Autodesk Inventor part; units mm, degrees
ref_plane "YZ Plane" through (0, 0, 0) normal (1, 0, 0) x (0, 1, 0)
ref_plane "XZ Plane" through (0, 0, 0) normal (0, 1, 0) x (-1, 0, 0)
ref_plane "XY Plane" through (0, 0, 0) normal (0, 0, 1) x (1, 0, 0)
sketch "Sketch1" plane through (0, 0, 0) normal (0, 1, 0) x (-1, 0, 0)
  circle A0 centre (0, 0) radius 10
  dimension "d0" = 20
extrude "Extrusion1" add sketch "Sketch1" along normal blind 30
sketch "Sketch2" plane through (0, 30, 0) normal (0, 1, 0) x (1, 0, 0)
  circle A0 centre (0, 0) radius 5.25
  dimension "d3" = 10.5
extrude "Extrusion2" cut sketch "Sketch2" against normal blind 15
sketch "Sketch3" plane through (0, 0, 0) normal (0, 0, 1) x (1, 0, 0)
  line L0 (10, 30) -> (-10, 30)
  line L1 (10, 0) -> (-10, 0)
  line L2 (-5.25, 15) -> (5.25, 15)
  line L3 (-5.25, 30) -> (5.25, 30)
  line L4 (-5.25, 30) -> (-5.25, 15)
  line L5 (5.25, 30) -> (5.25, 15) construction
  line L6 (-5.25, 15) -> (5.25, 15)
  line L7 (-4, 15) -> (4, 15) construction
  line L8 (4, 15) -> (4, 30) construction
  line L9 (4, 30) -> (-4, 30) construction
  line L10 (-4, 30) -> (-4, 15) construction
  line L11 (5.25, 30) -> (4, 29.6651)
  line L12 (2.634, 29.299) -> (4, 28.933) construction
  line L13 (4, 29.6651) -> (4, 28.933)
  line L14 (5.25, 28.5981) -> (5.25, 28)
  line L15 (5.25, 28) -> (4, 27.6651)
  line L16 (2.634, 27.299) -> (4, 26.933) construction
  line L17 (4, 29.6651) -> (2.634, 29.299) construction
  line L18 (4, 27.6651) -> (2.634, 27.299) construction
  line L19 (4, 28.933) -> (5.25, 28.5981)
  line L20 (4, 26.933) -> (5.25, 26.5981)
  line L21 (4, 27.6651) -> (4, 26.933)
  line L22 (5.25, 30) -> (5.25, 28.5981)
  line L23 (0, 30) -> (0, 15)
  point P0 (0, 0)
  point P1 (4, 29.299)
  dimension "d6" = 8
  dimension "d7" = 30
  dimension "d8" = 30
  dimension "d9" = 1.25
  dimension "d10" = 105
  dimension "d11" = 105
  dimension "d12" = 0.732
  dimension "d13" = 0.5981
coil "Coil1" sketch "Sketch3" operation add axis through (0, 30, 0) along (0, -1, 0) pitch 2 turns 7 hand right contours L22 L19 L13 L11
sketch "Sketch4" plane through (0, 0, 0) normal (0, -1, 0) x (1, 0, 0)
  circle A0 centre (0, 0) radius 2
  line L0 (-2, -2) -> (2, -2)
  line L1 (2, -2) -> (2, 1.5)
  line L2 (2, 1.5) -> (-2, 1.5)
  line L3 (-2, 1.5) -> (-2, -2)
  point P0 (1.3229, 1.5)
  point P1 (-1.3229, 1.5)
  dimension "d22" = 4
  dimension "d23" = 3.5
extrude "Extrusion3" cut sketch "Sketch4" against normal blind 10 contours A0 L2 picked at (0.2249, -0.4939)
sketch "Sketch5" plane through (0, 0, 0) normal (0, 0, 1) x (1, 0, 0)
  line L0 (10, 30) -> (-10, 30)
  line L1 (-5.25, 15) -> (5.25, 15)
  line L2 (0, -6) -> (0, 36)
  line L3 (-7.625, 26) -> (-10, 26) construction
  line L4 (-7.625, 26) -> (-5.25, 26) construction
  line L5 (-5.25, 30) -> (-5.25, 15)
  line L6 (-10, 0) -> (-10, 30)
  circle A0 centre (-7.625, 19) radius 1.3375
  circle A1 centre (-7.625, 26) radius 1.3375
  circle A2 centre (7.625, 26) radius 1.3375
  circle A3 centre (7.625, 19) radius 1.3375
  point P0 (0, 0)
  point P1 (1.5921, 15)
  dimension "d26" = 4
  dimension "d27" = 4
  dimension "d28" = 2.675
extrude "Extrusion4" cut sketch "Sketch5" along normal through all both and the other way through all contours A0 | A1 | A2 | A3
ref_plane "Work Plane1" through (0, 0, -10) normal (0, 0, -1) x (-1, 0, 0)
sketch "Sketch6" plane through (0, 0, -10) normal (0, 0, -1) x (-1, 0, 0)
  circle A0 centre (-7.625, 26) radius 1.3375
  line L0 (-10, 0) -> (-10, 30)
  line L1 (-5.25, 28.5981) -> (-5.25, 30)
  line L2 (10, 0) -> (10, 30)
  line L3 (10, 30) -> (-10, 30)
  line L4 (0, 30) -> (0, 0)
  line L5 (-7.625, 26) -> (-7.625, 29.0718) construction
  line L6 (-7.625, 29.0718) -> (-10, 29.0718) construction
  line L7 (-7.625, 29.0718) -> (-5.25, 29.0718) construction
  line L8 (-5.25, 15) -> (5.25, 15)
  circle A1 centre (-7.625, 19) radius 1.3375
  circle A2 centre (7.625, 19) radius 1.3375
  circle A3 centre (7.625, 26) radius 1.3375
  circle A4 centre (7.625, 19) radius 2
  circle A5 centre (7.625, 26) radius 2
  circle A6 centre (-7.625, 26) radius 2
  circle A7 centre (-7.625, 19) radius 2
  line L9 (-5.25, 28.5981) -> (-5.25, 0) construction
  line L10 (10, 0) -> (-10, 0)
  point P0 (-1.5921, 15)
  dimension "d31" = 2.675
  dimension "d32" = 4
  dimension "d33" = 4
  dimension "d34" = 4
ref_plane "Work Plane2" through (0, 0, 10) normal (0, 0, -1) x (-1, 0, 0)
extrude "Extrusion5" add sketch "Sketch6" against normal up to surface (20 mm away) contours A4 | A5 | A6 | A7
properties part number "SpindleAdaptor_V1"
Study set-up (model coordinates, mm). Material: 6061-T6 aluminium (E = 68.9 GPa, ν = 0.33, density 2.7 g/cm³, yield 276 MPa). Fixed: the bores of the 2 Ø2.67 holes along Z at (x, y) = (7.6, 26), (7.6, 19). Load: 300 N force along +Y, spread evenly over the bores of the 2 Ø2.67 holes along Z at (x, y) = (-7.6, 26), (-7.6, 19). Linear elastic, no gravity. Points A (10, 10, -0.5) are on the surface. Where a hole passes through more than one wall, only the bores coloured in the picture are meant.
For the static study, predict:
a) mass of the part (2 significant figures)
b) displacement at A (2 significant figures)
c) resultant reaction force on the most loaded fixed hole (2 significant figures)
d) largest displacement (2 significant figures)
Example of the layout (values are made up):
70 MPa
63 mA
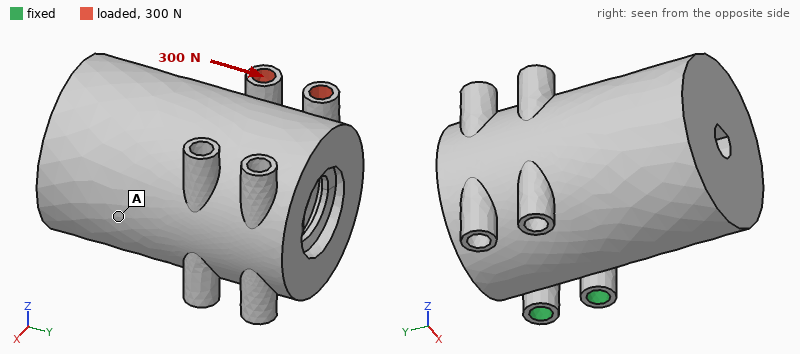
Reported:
22 g
12 µm
830 N
31 µm
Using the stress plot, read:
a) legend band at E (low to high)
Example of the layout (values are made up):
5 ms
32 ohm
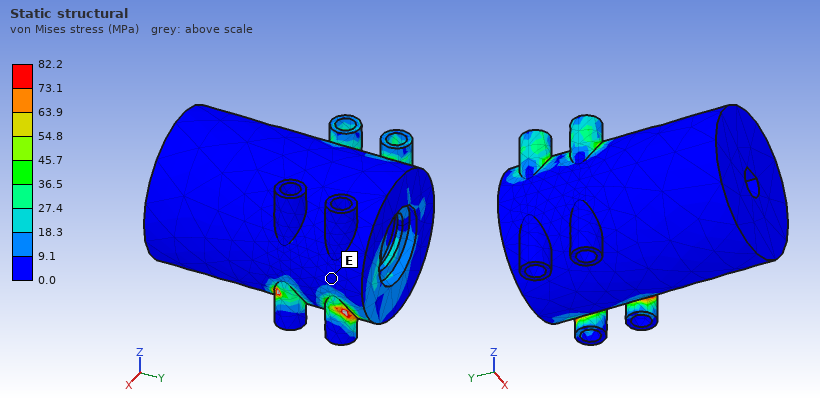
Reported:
0.0 to 9.1 MPa
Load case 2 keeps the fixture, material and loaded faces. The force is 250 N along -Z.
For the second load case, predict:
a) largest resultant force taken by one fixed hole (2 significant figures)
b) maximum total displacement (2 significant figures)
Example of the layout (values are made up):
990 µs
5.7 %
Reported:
130 N
59 µm
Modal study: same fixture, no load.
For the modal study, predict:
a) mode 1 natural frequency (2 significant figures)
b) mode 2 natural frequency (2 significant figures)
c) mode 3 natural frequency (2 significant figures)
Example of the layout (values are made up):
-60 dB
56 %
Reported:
3200 Hz
5200 Hz
7300 Hz
